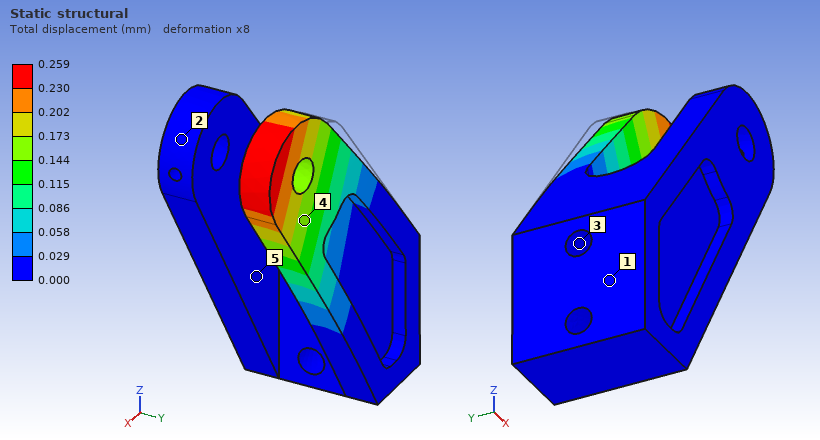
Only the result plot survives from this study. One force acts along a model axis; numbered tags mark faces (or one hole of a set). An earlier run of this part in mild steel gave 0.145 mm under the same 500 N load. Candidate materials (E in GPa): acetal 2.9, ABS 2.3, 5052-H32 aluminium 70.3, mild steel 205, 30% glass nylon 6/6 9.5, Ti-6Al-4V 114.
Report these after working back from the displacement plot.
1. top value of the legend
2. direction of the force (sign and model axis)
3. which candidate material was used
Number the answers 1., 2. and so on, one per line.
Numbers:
1. 0.259 mm
2. -Y
3. Ti-6Al-4V
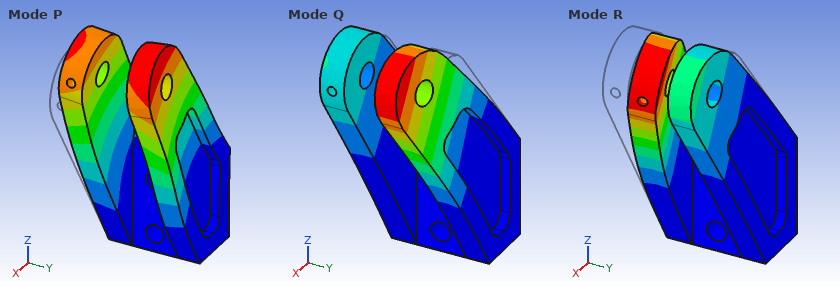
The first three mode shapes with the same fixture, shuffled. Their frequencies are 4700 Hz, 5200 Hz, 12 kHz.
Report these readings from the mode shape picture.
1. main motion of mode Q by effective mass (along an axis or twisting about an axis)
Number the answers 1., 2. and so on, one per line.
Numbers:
1. along Y
